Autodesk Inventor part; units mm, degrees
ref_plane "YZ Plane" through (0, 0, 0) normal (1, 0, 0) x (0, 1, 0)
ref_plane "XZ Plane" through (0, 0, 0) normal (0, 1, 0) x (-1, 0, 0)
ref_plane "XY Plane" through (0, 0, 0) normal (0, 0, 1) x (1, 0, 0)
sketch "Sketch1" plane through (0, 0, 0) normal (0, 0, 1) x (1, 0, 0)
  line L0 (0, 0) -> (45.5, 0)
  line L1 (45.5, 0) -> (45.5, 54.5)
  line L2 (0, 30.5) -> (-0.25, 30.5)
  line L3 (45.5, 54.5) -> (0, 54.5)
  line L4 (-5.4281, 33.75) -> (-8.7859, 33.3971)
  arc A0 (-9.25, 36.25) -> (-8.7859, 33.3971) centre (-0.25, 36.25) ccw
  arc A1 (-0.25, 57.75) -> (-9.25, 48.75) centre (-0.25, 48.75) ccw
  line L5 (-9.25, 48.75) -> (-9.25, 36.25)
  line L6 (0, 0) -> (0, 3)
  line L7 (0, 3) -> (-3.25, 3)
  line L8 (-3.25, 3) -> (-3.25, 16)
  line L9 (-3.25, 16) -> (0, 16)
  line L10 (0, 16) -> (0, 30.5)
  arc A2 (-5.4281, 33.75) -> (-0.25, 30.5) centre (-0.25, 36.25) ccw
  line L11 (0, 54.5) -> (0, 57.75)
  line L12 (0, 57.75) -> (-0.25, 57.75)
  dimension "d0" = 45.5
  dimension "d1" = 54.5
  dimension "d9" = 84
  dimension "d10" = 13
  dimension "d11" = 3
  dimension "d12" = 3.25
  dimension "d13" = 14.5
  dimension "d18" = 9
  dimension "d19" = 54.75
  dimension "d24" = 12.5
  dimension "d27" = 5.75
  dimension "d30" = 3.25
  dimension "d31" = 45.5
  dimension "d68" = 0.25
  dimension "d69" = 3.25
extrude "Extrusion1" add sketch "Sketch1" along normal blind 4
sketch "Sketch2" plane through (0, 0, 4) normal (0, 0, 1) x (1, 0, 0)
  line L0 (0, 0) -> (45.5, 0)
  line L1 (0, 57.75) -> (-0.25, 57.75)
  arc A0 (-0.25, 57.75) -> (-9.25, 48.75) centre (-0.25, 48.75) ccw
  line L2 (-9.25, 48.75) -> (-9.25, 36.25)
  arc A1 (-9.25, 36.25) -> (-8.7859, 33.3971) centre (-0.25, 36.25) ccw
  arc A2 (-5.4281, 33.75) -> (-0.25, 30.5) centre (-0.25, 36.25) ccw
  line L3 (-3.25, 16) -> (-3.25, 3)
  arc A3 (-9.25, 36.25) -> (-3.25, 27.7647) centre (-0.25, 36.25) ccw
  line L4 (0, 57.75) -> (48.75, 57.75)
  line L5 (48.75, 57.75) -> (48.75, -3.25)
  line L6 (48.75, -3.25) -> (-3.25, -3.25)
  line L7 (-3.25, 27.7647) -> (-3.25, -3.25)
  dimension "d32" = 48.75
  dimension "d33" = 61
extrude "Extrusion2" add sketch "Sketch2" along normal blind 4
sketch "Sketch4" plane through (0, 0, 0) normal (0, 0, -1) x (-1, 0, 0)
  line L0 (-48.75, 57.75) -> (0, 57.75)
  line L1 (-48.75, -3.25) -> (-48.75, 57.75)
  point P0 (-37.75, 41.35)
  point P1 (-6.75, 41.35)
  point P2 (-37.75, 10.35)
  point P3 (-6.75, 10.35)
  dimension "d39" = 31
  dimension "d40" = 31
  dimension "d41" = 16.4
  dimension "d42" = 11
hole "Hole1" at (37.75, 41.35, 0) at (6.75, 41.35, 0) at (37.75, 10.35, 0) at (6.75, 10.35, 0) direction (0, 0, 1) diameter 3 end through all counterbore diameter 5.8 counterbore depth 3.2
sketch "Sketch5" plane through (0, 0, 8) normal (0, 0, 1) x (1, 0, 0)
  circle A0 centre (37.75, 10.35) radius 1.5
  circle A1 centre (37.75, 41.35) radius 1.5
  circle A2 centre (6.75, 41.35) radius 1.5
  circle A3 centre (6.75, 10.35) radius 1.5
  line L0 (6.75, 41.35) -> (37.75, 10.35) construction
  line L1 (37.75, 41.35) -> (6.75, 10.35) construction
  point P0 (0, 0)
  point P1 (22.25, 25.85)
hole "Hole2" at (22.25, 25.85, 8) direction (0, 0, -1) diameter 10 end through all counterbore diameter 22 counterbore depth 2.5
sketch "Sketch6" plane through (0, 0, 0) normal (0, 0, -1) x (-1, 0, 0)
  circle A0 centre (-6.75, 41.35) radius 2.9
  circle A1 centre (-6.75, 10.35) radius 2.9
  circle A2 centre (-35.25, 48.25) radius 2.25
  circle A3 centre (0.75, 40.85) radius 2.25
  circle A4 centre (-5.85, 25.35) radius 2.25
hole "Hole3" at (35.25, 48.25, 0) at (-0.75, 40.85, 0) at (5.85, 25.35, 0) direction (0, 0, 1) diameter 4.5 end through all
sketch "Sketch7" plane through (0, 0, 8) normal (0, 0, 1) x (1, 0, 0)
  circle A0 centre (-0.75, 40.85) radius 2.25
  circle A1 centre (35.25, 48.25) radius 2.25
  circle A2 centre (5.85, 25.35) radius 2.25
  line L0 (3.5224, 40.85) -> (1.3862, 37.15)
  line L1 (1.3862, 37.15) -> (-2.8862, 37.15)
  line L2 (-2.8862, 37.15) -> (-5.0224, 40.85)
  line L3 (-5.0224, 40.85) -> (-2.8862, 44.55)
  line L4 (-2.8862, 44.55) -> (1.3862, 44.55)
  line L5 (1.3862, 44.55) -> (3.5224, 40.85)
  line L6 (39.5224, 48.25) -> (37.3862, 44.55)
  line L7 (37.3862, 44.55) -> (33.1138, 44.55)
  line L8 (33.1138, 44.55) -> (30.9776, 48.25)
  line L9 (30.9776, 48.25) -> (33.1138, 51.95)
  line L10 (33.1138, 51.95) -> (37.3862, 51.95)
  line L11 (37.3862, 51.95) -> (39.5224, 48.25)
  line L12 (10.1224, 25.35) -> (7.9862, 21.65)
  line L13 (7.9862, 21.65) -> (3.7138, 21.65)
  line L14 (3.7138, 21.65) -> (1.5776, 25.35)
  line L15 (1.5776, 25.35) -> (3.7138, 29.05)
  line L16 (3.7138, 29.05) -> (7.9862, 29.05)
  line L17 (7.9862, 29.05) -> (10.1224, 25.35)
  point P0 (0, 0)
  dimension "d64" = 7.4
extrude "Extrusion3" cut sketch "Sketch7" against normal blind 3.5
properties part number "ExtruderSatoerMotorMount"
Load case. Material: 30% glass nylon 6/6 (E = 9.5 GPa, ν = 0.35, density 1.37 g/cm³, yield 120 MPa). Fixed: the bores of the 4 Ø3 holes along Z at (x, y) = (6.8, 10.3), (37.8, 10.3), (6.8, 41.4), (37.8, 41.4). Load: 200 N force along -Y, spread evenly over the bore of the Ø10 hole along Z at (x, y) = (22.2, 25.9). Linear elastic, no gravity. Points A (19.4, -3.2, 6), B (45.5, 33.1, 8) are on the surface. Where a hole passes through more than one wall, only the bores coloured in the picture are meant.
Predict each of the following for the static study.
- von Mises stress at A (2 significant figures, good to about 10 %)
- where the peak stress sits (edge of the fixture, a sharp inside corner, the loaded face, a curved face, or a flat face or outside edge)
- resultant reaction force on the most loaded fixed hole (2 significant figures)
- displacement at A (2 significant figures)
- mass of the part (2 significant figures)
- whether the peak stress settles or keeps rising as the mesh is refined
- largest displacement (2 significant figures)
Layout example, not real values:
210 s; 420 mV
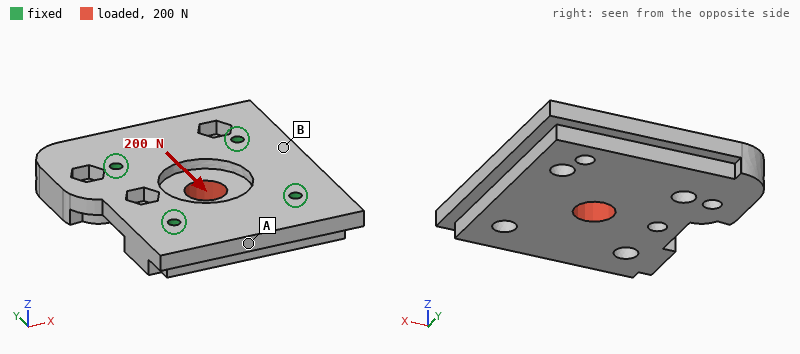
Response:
0.43 MPa; edge of the fixture; 54 N; 1.2 µm; 30 g; keeps rising; 2.3 µm
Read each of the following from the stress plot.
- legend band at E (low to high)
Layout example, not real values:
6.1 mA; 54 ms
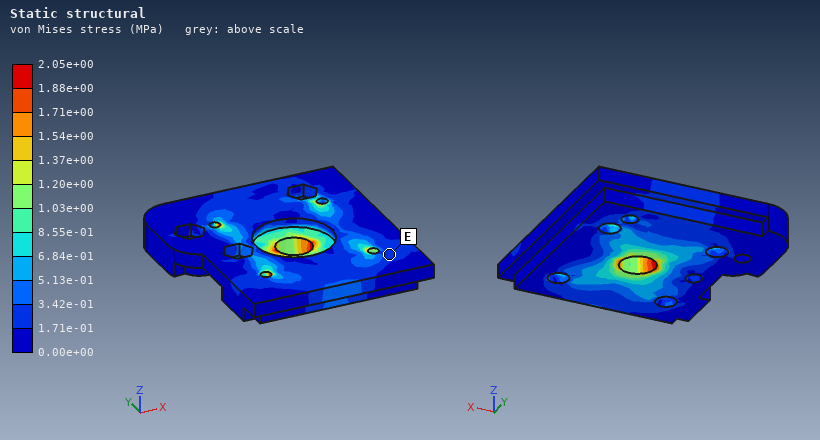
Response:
1.71e-01 to 3.42e-01 MPa
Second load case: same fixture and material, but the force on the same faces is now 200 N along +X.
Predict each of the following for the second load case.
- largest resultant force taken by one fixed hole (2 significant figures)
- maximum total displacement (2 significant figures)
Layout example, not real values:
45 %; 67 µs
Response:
54 N; 2.4 µm
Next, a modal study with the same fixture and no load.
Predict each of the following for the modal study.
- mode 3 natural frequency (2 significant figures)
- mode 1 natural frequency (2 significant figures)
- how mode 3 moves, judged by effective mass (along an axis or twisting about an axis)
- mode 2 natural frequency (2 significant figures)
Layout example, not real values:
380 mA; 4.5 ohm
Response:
9000 Hz; 6600 Hz; twisting about X; 7000 Hz
